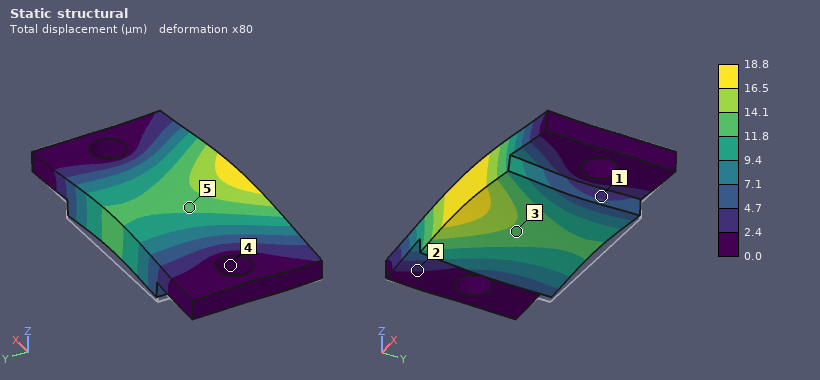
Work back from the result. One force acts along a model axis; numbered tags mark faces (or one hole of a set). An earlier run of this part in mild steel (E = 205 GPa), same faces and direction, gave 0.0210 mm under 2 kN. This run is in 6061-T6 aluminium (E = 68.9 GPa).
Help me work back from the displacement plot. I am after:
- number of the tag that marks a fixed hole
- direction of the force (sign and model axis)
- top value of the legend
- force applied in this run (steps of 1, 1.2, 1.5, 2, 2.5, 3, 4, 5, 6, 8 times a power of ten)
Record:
4
+Z
18.8 µm
600 N
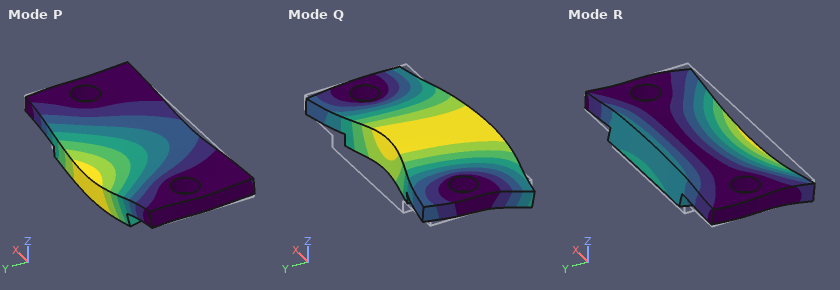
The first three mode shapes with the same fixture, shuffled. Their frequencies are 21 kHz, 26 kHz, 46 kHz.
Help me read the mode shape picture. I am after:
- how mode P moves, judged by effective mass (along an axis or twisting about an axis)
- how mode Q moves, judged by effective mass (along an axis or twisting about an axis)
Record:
along Z
along Y
